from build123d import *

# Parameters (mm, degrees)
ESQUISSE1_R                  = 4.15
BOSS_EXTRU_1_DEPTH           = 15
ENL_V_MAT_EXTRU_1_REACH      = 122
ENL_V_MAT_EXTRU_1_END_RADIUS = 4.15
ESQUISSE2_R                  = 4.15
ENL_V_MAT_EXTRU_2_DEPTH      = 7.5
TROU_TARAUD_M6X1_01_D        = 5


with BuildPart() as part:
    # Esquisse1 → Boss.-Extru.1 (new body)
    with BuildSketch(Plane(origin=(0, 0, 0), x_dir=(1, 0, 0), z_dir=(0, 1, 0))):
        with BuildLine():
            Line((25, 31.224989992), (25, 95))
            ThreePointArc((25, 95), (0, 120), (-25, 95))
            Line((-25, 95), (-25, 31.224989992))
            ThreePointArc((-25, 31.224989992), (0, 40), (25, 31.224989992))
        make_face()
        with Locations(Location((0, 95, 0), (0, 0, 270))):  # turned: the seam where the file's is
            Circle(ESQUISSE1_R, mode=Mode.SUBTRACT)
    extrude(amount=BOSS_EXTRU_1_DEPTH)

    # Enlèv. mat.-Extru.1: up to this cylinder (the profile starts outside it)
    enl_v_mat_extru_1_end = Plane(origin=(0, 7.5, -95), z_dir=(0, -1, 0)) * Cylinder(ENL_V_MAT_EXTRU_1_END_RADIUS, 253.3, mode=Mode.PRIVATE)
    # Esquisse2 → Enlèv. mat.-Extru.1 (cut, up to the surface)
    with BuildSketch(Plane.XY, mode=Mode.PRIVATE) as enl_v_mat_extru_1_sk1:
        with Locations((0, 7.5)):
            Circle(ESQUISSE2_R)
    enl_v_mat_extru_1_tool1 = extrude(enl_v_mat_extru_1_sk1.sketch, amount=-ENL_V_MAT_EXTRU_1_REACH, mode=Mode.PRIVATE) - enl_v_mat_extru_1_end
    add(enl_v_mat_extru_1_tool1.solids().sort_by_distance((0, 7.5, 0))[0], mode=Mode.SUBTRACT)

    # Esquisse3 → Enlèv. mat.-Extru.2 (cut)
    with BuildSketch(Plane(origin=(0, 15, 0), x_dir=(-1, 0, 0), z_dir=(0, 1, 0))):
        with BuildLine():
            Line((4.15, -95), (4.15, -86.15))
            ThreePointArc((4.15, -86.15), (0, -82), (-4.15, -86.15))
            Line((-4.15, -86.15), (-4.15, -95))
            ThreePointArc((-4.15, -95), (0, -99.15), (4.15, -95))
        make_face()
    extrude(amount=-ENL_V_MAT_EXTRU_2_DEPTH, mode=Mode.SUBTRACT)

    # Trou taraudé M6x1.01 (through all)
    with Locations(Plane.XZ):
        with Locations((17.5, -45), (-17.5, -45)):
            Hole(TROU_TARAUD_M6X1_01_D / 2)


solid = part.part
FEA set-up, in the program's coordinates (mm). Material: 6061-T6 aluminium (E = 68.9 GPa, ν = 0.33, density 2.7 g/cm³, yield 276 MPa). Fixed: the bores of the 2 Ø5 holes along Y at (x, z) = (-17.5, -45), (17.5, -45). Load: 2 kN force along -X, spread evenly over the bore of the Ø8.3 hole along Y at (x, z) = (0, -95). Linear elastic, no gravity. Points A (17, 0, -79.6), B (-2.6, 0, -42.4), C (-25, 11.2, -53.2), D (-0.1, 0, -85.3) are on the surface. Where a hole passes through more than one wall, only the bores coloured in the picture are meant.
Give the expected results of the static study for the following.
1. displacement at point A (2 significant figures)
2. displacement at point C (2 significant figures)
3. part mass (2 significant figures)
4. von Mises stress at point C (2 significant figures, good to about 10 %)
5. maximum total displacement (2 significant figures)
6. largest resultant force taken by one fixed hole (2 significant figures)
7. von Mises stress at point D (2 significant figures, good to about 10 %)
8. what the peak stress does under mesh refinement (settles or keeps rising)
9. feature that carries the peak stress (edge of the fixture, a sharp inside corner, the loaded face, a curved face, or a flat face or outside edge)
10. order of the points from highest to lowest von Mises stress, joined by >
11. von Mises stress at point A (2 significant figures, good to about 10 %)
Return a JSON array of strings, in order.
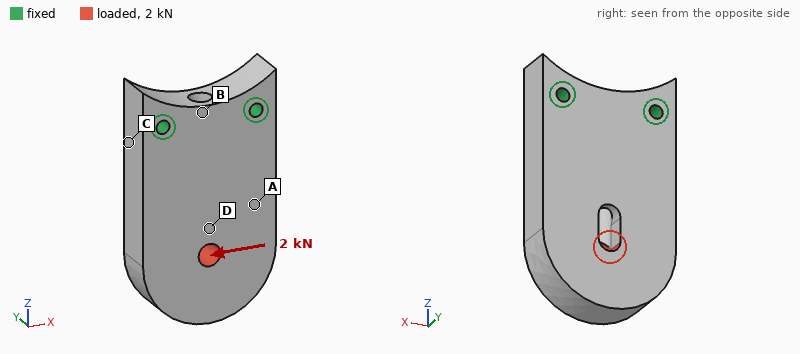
["11 µm", "3.7 µm", "140 g", "12 MPa", "24 µm", "2.9 kN", "17 MPa", "keeps rising", "edge of the fixture", "D > C > A > B", "6.6 MPa"]
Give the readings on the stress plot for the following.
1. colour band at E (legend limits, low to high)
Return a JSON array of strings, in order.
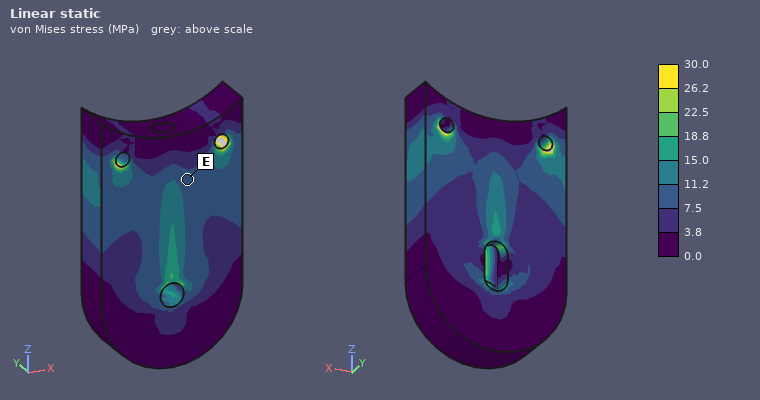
["7.5 to 11.2 MPa"]
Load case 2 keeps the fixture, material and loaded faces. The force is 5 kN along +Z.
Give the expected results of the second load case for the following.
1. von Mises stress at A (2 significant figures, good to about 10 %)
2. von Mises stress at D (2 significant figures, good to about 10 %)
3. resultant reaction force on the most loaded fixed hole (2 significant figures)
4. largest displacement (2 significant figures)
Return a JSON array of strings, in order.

["9.3 MPa", "18 MPa", "2.5 kN", "19 µm"]
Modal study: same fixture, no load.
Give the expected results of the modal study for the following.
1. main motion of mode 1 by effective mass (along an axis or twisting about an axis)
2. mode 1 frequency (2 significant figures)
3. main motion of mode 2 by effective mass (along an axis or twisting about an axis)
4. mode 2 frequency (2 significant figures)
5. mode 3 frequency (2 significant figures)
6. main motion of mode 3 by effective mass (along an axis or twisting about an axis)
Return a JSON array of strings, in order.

["along Y", "2200 Hz", "along X", "5900 Hz", "6900 Hz", "twisting about Z"]
